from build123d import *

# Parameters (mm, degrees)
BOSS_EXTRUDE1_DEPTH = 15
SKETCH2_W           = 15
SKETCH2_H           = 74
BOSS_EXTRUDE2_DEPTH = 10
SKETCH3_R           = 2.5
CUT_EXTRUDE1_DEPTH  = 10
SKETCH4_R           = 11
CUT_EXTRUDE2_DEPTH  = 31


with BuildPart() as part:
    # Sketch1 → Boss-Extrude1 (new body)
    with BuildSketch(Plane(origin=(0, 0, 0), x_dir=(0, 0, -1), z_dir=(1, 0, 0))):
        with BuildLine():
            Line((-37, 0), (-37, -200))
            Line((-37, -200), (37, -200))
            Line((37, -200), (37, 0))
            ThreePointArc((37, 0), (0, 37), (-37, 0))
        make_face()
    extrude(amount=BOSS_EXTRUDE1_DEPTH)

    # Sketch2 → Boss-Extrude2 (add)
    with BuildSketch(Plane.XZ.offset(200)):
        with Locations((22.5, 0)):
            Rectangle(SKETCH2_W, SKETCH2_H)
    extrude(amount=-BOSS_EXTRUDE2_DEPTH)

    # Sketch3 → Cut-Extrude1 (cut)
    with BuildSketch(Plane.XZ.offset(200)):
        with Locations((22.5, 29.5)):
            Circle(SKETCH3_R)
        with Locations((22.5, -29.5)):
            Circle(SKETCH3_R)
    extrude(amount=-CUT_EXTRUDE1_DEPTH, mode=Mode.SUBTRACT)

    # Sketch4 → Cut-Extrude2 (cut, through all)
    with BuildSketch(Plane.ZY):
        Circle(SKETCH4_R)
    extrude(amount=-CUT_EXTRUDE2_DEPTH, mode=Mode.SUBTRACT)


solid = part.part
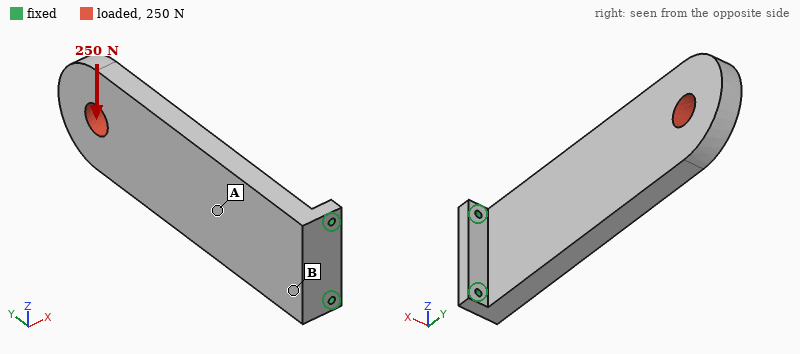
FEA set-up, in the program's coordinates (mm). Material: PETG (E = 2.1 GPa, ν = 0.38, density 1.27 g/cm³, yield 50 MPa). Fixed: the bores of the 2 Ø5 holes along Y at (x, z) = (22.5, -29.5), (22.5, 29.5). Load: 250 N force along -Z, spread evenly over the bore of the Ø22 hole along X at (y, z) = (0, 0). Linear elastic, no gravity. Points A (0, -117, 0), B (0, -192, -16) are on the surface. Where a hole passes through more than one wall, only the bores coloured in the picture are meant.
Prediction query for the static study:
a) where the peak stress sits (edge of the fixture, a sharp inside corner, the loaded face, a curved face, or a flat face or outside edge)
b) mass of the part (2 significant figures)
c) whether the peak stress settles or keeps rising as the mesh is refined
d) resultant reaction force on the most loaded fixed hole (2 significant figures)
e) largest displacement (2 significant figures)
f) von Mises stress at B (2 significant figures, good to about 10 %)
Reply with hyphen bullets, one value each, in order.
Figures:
- edge of the fixture
- 330 g
- keeps rising
- 820 N
- 2.0 mm
- 3.7 MPa
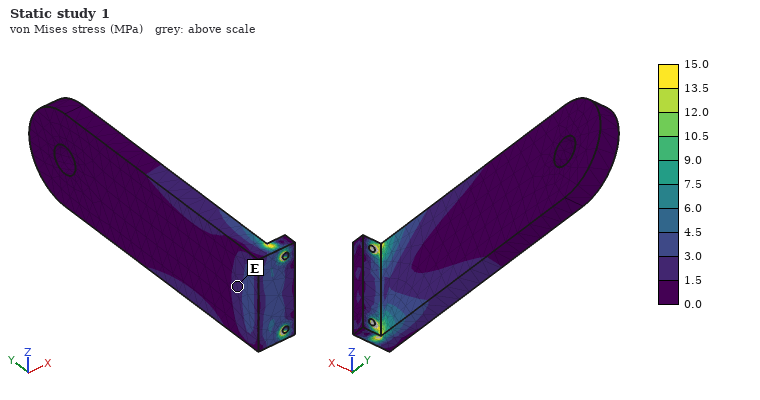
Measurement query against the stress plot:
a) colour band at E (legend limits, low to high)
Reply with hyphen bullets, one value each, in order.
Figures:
- 1.5 to 3.0 MPa
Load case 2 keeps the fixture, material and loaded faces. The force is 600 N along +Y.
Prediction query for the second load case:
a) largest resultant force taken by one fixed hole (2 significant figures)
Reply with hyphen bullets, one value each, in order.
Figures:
- 300 N
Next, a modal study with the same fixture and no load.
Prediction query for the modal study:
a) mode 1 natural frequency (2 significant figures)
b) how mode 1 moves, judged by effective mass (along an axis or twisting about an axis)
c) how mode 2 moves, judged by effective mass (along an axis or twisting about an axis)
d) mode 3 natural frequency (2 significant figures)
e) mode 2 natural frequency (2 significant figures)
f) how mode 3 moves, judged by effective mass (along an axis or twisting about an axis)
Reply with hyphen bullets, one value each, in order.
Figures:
- 44 Hz
- along X
- along Z
- 300 Hz
- 180 Hz
- along X
